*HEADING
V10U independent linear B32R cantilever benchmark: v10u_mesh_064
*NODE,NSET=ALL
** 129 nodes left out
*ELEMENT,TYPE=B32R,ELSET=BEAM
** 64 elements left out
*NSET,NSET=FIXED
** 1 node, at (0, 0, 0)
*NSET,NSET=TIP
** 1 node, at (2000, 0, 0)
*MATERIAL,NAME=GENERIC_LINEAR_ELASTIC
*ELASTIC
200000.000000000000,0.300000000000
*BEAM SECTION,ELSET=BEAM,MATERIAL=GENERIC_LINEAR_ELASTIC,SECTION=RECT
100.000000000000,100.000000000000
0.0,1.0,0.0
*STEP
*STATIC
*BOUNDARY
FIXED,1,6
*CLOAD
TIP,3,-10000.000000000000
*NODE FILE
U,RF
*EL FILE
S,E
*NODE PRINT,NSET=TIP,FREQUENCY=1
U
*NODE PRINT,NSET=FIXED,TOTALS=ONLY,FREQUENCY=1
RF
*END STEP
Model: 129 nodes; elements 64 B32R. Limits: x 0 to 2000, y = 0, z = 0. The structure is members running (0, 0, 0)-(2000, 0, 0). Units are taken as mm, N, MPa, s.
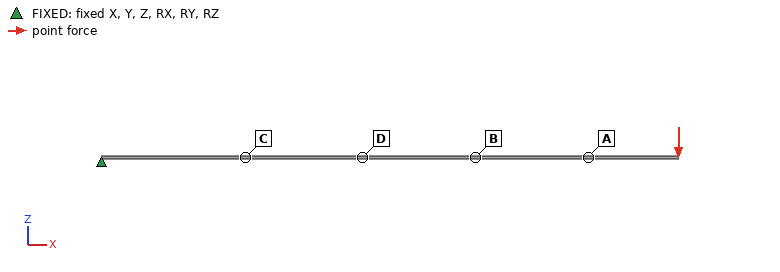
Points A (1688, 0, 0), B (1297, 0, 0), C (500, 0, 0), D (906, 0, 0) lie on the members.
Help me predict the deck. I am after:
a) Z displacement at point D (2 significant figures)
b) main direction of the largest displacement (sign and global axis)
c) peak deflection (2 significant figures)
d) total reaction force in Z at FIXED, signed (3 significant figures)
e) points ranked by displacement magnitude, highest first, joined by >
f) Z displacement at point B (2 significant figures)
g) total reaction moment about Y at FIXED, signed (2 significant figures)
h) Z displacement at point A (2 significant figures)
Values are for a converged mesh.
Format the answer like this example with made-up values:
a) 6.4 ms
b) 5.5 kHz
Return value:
a) -4.2 mm
b) -Z
c) 16 mm
d) 10000 N
e) A > B > D > C
f) -7.9 mm
g) -2.0e+07 N·mm
h) -12 mm
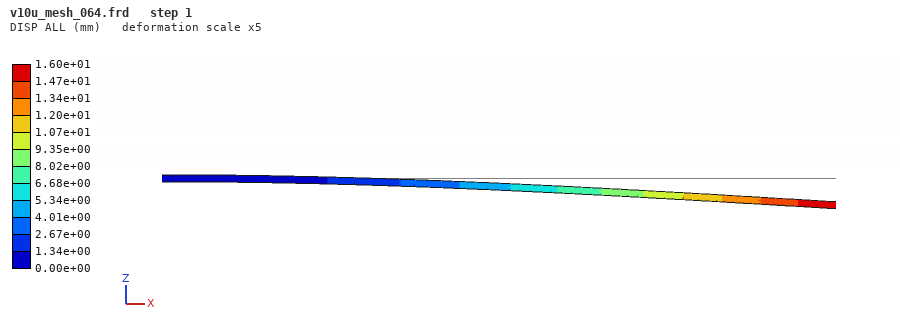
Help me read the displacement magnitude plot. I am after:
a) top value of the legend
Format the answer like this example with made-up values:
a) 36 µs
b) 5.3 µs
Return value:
a) 1.60e+01 mm
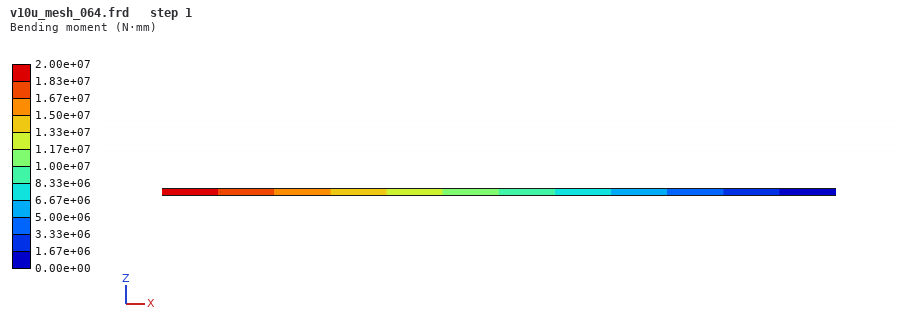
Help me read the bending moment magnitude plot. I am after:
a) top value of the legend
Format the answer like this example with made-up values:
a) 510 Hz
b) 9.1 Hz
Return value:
a) 2.00e+07 N·mm
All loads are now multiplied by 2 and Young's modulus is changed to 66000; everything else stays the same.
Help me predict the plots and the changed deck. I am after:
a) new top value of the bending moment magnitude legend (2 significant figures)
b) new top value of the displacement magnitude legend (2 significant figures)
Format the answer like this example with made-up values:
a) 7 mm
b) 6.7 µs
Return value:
a) 4.0e+07 N·mm
b) 97 mm
